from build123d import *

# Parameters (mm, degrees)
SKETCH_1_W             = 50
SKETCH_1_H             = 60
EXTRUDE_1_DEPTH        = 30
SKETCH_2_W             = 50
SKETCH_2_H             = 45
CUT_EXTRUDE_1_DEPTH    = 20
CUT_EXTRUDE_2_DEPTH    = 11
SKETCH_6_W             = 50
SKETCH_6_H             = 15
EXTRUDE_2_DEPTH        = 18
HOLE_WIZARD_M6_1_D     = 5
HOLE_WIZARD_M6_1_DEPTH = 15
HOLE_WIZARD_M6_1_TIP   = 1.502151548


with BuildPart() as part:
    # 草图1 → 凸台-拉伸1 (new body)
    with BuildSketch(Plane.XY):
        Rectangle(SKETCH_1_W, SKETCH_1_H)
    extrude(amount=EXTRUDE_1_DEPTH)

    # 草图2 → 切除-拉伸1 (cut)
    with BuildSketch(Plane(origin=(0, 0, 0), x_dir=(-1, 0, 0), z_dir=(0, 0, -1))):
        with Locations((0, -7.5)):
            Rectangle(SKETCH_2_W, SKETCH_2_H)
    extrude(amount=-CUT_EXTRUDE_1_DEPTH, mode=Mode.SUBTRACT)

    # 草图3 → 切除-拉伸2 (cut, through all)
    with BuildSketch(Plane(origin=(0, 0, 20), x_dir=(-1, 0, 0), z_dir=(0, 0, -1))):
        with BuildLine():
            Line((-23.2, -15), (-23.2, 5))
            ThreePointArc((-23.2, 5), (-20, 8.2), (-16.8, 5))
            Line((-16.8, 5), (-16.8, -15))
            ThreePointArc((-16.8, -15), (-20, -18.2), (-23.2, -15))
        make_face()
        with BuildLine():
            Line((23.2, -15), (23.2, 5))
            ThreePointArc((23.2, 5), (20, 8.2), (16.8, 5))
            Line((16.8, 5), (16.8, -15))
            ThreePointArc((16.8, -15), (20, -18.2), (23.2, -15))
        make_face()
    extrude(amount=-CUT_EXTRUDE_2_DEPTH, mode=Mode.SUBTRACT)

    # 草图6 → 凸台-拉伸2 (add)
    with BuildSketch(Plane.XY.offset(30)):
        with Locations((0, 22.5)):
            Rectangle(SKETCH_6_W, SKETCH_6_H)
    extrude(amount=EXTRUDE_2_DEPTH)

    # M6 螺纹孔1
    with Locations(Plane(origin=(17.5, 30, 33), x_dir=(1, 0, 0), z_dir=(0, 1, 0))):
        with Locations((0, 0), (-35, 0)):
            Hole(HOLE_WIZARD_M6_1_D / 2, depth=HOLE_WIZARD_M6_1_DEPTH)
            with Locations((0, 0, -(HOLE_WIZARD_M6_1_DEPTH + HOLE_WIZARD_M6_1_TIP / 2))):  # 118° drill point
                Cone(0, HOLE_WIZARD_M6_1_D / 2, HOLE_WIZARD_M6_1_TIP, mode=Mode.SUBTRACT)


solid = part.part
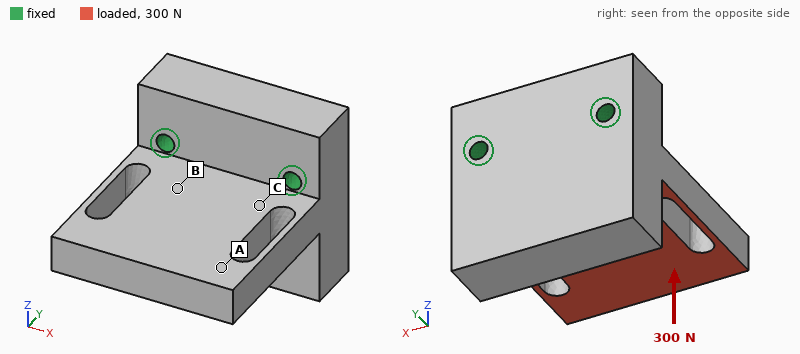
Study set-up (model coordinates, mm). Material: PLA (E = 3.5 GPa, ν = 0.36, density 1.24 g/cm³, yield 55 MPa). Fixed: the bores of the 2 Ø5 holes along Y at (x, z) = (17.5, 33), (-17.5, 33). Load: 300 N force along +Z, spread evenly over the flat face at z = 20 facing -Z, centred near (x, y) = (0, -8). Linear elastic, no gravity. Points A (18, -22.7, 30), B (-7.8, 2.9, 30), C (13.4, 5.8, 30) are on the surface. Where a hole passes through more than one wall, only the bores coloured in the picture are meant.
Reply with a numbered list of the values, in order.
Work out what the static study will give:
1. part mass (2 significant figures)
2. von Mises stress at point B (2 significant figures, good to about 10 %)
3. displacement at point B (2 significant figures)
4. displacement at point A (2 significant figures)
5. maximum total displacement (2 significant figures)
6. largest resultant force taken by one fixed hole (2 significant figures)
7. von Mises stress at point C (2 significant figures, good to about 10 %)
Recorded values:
1. 68 g
2. 5.4 MPa
3. 0.098 mm
4. 0.37 mm
5. 0.47 mm
6. 160 N
7. 6.4 MPa
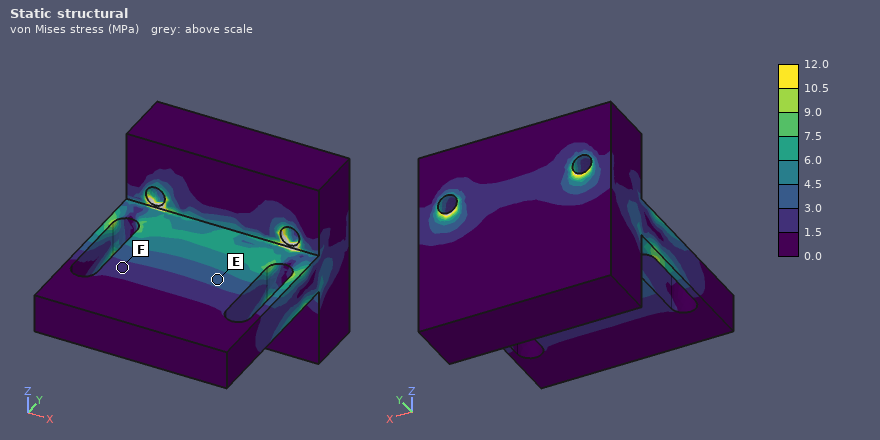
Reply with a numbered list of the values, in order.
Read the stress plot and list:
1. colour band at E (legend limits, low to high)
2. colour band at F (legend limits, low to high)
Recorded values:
1. 3.0 to 4.5 MPa
2. 1.5 to 3.0 MPa
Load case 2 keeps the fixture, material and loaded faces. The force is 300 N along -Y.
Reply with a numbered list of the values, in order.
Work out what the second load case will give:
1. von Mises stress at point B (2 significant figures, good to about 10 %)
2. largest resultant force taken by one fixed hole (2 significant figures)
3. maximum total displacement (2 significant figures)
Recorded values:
1. 1.1 MPa
2. 150 N
3. 0.14 mm
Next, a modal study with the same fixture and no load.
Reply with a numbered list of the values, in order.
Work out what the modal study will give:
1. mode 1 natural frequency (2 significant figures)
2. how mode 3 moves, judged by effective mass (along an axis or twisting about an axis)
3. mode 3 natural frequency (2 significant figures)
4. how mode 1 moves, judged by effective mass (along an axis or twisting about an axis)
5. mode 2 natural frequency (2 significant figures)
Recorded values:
1. 990 Hz
2. along X
3. 2700 Hz
4. along Z
5. 2200 Hz
